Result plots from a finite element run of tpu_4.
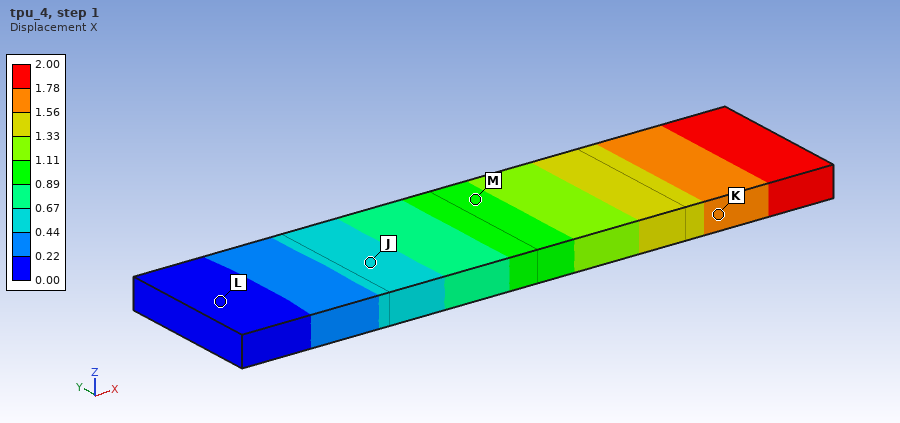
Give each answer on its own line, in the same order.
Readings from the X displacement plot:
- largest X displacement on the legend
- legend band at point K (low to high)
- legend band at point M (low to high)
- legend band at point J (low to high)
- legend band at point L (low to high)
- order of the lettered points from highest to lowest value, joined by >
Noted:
2.00
1.56 to 1.78
0.89 to 1.11
0.44 to 0.67
0.00 to 0.22
K > M > J > L
